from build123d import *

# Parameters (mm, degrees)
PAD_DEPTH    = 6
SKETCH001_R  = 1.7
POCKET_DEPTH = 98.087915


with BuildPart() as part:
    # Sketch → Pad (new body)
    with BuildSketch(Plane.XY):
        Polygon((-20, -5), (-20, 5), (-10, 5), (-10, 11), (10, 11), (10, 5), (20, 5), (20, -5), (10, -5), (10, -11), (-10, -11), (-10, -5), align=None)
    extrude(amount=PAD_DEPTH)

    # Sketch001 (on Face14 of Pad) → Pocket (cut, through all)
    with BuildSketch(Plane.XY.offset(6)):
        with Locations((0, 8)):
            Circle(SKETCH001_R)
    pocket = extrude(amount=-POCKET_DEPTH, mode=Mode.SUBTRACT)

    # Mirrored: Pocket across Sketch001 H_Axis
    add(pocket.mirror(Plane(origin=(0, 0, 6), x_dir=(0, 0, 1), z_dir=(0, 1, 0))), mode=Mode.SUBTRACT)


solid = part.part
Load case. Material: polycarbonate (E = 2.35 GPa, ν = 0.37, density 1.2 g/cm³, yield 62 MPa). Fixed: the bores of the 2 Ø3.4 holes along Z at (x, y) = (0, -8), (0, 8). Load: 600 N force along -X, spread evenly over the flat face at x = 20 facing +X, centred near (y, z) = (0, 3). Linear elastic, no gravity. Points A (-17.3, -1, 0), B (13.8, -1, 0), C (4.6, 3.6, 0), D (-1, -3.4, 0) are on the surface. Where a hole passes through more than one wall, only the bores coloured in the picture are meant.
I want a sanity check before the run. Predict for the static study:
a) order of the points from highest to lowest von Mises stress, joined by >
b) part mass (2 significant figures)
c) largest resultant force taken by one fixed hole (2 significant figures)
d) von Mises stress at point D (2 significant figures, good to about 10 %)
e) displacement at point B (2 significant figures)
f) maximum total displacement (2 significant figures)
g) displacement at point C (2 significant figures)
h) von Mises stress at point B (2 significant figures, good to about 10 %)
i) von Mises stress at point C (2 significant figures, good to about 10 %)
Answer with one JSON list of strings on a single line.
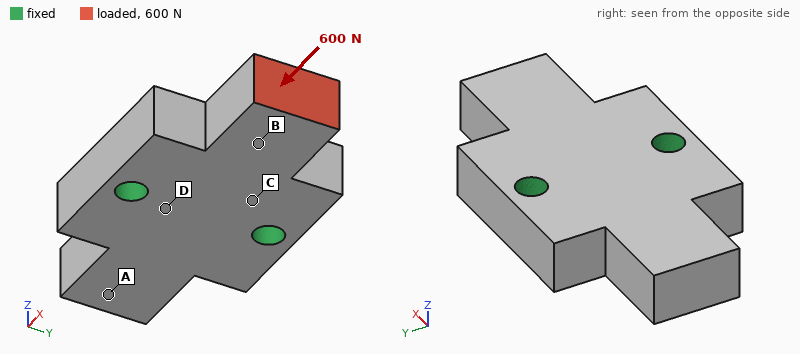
["B > C > D > A", "4.5 g", "310 N", "3.0 MPa", "51 µm", "77 µm", "19 µm", "9.3 MPa", "6.9 MPa"]
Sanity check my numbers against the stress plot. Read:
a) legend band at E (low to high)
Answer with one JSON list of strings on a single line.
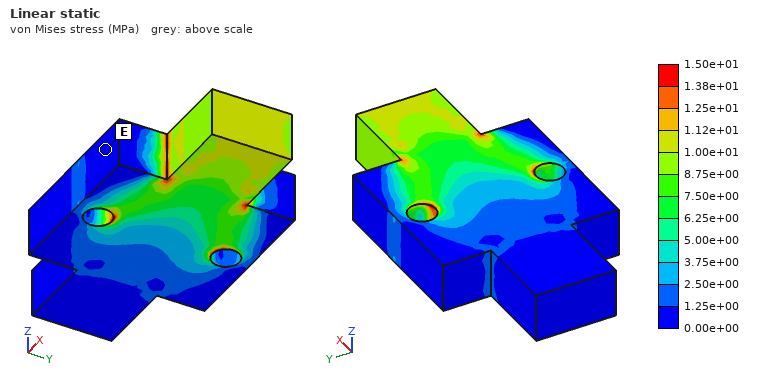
["0.00e+00 to 1.25e+00 MPa"]
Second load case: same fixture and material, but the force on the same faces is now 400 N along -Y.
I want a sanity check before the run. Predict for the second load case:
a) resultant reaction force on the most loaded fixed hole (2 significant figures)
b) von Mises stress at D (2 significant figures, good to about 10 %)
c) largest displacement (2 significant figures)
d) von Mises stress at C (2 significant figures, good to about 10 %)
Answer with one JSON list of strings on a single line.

["500 N", "2.5 MPa", "0.43 mm", "11 MPa"]
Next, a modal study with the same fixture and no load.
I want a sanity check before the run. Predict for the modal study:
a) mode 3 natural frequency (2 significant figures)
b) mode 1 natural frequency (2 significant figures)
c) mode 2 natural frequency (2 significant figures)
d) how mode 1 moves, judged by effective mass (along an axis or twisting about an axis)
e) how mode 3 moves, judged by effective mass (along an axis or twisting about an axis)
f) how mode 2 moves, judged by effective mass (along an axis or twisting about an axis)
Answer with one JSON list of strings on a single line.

["9000 Hz", "3700 Hz", "4200 Hz", "twisting about Y", "twisting about Z", "along Z"]
